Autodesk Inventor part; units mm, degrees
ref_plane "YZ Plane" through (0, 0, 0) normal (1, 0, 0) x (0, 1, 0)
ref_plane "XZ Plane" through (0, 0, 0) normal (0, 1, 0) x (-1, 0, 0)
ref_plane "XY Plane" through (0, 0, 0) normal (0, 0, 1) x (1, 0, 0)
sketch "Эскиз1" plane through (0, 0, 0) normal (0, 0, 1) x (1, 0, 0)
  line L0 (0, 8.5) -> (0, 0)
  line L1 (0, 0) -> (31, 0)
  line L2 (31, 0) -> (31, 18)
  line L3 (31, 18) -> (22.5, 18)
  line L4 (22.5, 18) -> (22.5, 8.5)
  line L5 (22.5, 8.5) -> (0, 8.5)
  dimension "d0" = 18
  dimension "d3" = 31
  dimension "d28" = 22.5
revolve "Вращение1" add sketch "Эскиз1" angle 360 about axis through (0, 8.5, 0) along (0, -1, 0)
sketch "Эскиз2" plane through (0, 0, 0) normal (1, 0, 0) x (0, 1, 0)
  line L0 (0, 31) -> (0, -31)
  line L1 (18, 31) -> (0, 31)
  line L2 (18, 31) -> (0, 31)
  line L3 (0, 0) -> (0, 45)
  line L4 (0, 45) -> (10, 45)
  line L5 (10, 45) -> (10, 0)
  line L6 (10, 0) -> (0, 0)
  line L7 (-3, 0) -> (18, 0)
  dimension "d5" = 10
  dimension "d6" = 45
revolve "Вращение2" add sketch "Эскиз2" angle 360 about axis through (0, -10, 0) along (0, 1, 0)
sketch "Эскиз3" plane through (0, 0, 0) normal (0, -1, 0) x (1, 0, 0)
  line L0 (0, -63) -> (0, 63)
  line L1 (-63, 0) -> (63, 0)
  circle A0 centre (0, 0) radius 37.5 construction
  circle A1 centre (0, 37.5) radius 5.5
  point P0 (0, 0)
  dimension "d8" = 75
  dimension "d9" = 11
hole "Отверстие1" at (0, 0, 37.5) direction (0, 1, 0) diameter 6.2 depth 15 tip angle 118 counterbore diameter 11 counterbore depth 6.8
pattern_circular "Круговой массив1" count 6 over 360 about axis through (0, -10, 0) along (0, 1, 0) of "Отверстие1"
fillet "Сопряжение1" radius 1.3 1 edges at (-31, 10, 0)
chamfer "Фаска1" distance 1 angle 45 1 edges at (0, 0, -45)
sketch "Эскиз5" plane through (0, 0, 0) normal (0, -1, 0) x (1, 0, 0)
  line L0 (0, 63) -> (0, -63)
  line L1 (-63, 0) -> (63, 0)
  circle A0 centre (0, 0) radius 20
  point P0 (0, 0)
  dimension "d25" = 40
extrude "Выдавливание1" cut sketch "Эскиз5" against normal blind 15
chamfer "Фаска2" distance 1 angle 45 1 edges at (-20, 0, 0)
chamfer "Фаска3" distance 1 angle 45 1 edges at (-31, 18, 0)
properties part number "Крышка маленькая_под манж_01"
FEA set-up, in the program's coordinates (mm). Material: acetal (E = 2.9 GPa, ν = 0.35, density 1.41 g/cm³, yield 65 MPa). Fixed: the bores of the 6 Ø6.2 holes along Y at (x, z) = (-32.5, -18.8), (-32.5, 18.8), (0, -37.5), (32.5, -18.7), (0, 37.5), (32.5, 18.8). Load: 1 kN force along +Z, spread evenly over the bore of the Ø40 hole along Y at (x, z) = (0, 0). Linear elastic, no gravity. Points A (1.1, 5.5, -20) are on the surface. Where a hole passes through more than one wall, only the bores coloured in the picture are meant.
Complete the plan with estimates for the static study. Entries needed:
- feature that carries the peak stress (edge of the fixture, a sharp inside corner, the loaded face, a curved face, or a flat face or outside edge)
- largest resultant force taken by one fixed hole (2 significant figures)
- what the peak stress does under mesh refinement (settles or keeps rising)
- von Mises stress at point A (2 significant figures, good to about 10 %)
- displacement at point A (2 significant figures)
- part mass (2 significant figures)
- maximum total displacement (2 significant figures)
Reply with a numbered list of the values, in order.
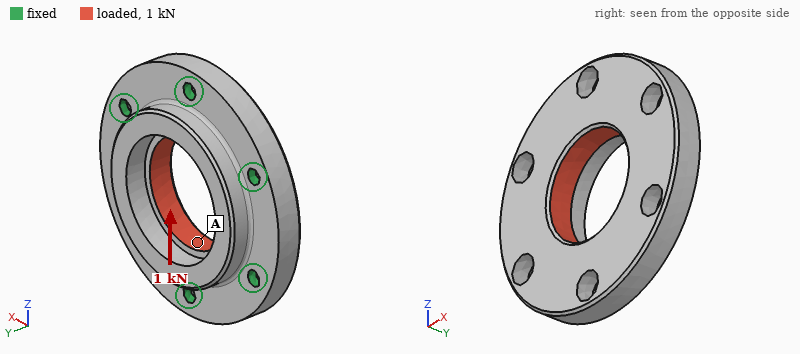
1. edge of the fixture
2. 210 N
3. keeps rising
4. 0.91 MPa
5. 14 µm
6. 81 g
7. 16 µm
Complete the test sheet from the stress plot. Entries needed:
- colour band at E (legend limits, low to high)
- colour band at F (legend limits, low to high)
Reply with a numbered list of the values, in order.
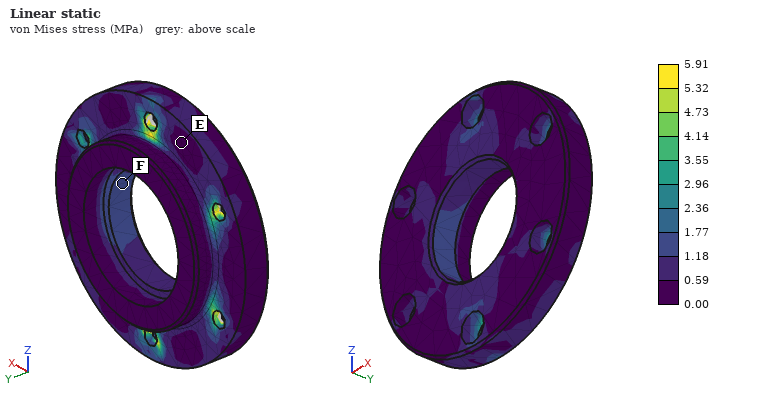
1. 0.00 to 0.59 MPa
2. 1.18 to 1.77 MPa
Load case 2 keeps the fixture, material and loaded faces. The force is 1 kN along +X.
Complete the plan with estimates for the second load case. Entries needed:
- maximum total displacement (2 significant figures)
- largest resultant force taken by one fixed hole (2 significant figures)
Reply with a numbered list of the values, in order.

1. 17 µm
2. 190 N
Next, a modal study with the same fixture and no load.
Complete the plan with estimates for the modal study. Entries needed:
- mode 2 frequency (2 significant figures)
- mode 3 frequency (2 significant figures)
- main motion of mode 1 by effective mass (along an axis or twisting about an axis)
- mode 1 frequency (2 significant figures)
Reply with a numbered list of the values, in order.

1. 4900 Hz
2. 4900 Hz
3. along Y
4. 3800 Hz
